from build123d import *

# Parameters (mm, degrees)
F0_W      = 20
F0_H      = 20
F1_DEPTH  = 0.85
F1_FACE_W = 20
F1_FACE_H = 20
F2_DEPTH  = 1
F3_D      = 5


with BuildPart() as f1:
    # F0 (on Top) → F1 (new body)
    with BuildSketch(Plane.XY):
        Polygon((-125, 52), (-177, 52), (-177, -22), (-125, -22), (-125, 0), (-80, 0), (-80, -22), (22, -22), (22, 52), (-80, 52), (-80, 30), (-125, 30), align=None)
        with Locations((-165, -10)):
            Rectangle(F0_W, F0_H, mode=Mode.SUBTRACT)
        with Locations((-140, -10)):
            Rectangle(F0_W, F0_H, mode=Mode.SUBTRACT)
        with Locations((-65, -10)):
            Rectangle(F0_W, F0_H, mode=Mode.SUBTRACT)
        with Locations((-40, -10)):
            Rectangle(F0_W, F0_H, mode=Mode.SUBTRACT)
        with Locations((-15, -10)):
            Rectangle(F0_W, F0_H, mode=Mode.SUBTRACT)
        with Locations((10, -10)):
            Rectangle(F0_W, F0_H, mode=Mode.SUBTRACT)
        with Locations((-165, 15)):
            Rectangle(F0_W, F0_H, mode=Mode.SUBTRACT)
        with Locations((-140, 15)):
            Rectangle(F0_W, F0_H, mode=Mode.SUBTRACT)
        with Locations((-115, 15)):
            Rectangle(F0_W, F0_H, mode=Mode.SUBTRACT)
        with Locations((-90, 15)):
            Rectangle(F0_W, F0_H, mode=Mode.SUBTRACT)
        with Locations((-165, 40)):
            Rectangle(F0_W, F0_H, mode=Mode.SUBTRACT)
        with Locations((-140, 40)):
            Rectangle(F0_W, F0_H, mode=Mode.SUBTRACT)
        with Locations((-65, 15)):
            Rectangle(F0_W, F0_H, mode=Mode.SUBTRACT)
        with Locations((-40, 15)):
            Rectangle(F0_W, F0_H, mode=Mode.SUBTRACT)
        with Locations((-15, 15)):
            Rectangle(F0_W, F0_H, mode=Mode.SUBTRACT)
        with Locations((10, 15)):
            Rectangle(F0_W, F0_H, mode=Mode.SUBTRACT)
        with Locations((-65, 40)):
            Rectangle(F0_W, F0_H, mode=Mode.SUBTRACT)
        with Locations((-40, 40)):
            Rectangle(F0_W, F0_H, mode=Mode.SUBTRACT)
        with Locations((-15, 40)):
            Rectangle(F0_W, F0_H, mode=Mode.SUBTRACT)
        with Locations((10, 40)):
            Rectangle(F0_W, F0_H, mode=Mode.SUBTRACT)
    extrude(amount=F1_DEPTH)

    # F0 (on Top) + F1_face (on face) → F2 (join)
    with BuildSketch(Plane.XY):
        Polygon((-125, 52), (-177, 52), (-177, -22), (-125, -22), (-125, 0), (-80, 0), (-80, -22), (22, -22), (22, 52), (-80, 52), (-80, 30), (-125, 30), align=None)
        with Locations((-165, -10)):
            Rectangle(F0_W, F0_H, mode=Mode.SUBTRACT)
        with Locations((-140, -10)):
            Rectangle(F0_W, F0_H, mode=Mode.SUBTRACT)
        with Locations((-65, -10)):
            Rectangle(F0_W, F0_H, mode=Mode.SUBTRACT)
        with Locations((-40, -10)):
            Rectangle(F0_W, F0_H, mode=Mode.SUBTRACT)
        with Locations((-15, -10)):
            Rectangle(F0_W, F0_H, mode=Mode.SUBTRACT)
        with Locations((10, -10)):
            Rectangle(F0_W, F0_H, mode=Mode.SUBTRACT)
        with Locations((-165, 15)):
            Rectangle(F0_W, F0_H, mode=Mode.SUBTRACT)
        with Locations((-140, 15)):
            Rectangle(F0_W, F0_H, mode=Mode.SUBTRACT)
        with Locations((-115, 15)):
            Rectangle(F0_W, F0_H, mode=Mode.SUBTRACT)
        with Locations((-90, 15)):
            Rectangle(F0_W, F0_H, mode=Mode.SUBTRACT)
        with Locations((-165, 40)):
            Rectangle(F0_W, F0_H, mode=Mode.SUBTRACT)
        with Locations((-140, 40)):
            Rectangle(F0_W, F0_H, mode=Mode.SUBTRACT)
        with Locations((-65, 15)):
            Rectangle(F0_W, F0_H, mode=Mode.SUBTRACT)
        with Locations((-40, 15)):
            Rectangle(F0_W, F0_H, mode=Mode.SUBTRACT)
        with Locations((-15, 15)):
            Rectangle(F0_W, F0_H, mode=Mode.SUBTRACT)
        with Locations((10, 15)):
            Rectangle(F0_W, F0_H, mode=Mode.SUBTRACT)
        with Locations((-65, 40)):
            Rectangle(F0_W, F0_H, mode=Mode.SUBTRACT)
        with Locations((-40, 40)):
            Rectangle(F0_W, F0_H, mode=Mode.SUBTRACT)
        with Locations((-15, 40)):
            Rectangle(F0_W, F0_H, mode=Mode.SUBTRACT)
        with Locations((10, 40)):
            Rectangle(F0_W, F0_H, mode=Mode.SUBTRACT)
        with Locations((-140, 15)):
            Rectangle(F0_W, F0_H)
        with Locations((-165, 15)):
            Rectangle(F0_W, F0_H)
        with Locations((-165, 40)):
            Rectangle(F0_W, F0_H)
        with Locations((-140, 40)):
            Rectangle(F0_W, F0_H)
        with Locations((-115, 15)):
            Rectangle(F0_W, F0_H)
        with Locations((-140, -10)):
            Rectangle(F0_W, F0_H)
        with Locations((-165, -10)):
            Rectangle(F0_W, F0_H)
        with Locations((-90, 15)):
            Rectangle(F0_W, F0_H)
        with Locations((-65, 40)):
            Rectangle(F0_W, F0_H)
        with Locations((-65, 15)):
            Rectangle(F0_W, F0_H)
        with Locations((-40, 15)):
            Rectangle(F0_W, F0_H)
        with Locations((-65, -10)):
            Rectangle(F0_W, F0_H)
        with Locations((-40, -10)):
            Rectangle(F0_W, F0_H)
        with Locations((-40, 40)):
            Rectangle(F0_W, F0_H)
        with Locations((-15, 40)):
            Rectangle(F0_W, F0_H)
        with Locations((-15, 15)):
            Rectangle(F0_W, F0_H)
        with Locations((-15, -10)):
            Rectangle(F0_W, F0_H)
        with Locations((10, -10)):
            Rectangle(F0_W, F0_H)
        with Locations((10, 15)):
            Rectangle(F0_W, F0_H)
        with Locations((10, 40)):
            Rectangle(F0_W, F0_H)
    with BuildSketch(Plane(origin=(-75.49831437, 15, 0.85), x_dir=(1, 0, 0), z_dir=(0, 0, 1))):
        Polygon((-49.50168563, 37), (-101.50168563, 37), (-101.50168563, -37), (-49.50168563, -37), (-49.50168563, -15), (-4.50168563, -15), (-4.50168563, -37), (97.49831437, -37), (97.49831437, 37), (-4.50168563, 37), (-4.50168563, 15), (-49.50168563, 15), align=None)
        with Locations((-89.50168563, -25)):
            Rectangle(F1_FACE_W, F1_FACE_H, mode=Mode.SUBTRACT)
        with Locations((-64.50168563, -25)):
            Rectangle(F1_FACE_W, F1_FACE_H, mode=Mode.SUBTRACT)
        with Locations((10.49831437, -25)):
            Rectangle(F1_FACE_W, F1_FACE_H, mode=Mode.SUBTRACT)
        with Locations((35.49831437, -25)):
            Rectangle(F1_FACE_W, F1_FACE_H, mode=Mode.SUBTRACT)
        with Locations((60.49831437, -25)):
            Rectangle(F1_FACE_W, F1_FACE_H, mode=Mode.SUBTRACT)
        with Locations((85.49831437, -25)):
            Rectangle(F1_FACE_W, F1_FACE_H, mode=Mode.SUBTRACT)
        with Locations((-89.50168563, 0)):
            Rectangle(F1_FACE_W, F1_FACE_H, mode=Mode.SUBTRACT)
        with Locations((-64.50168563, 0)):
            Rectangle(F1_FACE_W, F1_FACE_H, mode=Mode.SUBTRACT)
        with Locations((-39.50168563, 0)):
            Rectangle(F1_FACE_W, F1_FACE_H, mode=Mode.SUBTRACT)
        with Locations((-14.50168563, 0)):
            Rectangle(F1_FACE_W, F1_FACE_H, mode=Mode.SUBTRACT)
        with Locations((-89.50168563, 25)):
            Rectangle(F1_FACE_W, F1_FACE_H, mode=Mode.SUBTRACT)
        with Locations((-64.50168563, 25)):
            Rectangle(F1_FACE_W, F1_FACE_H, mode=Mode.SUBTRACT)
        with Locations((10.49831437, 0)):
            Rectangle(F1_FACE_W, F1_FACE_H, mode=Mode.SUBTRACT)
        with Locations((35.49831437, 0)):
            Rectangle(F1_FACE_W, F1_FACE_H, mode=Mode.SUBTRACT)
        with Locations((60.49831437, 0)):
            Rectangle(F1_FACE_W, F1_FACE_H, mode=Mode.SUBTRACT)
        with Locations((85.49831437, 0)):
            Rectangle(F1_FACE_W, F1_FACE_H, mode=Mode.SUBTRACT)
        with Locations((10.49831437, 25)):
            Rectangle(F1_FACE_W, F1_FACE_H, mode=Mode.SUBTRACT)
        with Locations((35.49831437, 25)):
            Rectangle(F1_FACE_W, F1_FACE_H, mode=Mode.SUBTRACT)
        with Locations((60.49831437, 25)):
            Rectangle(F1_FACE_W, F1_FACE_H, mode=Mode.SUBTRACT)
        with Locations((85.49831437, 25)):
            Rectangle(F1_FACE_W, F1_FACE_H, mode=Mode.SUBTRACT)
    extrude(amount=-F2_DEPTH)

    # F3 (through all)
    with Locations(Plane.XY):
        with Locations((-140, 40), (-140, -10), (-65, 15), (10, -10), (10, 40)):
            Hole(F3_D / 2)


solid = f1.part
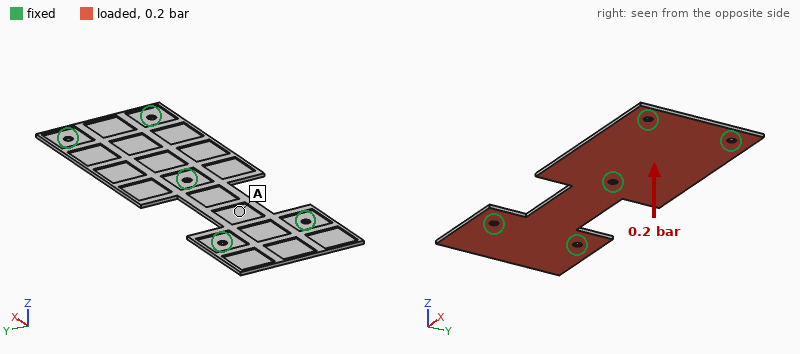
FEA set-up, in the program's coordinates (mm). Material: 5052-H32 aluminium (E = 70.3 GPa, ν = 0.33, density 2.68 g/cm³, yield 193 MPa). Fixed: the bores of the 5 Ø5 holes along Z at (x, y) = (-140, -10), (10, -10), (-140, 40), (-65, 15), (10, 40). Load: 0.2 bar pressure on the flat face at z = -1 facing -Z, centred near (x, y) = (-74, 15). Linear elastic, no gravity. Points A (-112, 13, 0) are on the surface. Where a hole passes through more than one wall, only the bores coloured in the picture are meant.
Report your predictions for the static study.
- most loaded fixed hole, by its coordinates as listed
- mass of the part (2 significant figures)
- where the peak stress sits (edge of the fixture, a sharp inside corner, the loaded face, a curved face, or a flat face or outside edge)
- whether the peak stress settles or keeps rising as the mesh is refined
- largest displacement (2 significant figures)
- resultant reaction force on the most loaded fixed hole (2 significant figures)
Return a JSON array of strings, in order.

["(-65, 15)", "45 g", "edge of the fixture", "keeps rising", "0.41 mm", "110 N"]
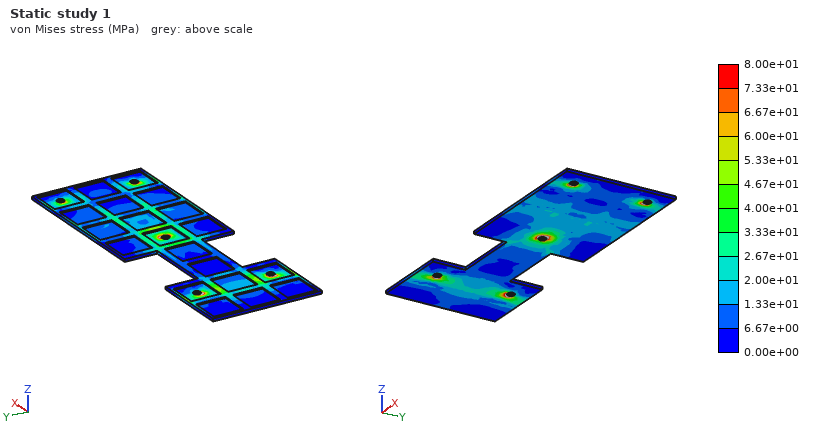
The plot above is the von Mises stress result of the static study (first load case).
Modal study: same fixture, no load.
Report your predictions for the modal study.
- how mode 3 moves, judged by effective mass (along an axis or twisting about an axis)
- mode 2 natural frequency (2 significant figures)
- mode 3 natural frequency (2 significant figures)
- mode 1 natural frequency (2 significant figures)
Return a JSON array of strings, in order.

["along Z", "740 Hz", "910 Hz", "710 Hz"]
